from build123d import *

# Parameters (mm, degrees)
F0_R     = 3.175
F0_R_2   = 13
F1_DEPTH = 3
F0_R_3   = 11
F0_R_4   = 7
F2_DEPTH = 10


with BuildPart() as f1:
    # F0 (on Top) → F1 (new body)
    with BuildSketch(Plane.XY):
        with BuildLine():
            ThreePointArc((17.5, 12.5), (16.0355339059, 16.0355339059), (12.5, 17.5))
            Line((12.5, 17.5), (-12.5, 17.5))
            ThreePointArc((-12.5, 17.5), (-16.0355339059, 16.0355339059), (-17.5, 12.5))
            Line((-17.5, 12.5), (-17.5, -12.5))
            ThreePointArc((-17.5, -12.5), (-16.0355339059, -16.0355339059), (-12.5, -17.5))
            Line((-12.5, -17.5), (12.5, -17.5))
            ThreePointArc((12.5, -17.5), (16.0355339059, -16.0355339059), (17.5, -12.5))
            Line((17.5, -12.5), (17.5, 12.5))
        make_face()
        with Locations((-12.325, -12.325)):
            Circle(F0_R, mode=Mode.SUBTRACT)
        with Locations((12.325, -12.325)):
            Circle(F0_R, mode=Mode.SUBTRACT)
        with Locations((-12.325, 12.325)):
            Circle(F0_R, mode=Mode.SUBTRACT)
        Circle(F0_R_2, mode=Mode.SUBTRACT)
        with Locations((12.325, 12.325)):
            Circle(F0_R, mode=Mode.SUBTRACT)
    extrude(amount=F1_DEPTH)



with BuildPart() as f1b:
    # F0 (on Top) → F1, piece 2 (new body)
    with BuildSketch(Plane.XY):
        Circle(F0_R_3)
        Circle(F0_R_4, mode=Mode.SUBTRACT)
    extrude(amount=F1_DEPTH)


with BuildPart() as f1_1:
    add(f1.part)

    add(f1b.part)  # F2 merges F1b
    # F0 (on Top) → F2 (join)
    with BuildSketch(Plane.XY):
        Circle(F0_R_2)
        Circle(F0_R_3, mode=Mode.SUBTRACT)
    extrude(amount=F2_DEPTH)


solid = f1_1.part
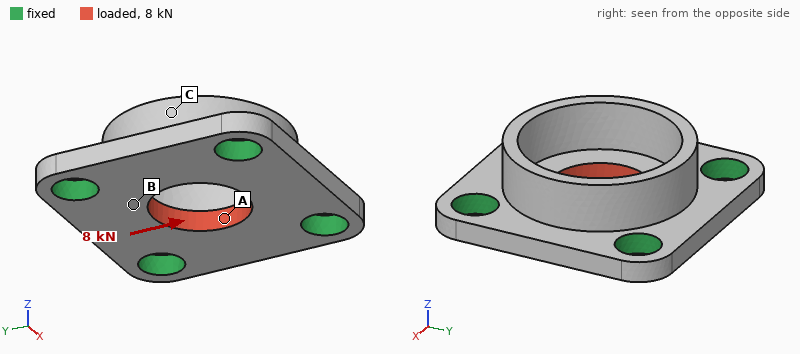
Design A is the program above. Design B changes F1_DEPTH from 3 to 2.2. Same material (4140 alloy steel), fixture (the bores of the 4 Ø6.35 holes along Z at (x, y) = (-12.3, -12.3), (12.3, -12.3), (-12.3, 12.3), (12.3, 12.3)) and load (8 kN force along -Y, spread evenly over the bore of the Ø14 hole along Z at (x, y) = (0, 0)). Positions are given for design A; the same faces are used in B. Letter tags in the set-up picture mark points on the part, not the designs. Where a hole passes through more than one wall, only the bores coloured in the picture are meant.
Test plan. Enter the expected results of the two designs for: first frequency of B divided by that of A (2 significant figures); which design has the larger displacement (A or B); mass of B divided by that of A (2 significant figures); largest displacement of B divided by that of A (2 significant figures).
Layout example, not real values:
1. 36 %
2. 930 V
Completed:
1. 0.80
2. B
3. 0.84
4. 1.4
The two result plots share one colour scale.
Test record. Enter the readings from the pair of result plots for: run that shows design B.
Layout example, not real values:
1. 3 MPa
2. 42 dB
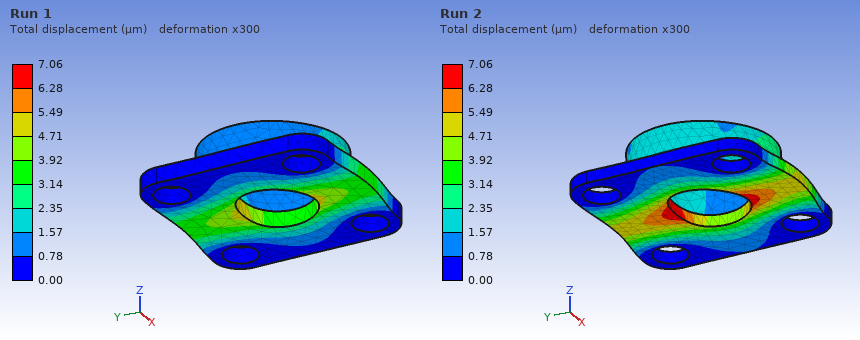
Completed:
1. Run 2
